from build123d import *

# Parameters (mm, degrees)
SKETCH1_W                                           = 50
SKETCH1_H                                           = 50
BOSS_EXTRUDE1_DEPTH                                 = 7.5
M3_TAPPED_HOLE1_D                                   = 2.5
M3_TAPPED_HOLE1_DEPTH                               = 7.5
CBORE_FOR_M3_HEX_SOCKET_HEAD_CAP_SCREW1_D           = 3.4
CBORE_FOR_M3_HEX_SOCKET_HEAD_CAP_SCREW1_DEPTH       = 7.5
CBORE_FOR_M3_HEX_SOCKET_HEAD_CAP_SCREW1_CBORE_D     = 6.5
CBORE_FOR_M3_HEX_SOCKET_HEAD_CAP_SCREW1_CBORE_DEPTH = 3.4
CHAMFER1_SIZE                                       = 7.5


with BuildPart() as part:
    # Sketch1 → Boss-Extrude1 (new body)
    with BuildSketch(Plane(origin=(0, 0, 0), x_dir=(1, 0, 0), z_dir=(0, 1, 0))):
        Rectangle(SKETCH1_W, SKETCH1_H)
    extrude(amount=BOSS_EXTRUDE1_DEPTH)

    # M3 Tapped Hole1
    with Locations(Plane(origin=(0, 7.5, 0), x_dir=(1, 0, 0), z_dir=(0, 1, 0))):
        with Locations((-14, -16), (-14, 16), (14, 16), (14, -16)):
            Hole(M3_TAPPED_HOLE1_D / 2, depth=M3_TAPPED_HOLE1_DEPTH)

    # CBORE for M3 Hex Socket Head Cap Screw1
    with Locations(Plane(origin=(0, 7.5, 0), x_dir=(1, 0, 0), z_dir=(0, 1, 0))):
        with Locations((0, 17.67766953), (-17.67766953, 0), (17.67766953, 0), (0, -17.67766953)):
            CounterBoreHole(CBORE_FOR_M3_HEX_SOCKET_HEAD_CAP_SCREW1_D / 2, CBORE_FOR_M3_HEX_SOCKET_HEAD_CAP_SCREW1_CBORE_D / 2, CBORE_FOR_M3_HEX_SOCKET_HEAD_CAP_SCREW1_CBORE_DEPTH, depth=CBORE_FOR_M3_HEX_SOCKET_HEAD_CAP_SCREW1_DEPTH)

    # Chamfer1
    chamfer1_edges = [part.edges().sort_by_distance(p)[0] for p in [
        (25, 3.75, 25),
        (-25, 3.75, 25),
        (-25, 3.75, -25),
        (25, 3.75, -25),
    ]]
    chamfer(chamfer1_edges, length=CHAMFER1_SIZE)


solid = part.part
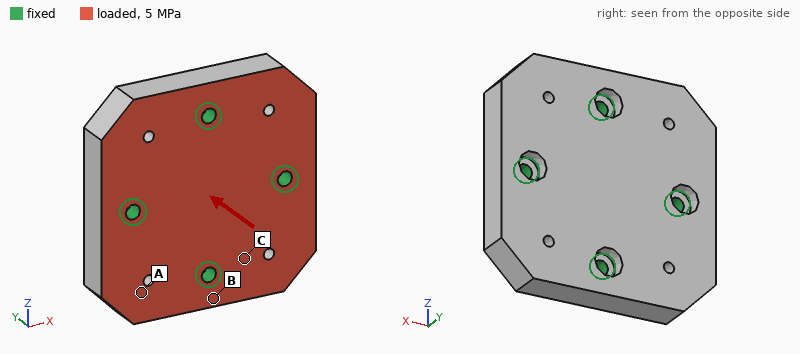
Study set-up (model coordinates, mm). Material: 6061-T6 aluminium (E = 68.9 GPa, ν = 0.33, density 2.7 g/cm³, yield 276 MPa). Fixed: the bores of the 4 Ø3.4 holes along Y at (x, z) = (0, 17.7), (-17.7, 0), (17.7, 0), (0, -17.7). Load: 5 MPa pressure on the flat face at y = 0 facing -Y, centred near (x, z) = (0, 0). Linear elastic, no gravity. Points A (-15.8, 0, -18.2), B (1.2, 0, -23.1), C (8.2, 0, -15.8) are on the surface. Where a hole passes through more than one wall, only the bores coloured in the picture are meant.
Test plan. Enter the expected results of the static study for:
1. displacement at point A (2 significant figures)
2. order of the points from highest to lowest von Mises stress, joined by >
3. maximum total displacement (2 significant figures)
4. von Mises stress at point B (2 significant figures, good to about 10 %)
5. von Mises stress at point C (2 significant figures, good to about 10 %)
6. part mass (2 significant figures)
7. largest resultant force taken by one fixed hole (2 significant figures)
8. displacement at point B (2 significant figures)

22 µm
B > C > A
32 µm
57 MPa
27 MPa
46 g
2.9 kN
6.7 µm
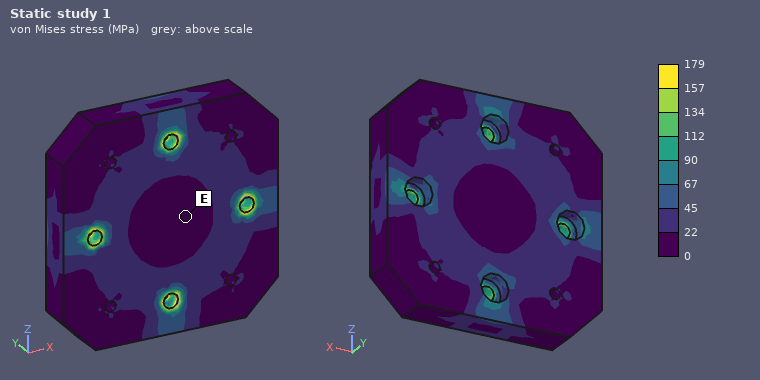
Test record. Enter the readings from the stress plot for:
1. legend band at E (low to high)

0 to 22 MPa
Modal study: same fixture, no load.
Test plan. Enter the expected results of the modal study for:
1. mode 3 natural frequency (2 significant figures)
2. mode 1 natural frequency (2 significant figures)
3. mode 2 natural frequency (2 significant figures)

15 kHz
14 kHz
15 kHz
